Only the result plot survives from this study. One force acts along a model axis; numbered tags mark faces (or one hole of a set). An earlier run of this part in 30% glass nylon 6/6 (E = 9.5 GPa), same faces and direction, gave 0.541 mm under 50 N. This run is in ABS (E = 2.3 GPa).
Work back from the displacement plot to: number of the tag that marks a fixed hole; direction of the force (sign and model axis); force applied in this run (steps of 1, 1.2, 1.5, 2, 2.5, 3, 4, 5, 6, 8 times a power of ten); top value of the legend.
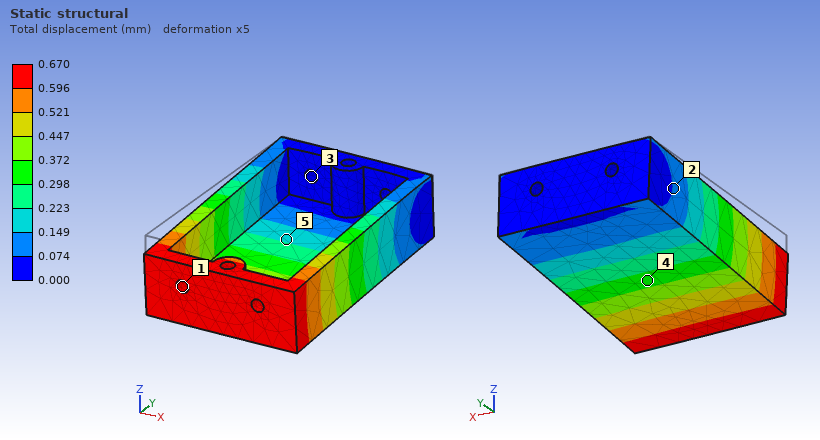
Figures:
3
-Z
15 N
0.670 mm
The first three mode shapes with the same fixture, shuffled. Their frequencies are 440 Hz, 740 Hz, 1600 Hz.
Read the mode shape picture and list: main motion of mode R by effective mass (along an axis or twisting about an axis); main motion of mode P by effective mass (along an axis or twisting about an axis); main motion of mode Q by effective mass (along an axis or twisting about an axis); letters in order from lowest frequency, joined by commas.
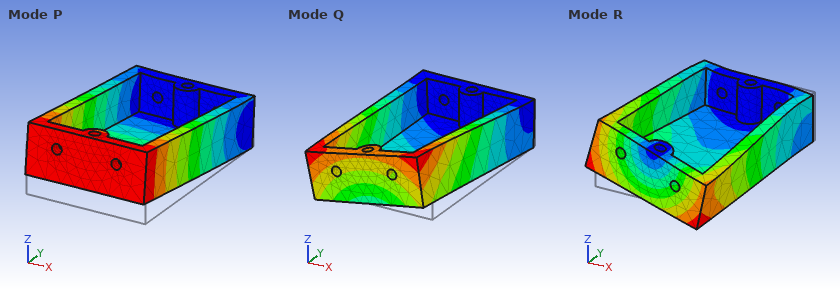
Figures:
along X
along Z
along X
P, Q, R
